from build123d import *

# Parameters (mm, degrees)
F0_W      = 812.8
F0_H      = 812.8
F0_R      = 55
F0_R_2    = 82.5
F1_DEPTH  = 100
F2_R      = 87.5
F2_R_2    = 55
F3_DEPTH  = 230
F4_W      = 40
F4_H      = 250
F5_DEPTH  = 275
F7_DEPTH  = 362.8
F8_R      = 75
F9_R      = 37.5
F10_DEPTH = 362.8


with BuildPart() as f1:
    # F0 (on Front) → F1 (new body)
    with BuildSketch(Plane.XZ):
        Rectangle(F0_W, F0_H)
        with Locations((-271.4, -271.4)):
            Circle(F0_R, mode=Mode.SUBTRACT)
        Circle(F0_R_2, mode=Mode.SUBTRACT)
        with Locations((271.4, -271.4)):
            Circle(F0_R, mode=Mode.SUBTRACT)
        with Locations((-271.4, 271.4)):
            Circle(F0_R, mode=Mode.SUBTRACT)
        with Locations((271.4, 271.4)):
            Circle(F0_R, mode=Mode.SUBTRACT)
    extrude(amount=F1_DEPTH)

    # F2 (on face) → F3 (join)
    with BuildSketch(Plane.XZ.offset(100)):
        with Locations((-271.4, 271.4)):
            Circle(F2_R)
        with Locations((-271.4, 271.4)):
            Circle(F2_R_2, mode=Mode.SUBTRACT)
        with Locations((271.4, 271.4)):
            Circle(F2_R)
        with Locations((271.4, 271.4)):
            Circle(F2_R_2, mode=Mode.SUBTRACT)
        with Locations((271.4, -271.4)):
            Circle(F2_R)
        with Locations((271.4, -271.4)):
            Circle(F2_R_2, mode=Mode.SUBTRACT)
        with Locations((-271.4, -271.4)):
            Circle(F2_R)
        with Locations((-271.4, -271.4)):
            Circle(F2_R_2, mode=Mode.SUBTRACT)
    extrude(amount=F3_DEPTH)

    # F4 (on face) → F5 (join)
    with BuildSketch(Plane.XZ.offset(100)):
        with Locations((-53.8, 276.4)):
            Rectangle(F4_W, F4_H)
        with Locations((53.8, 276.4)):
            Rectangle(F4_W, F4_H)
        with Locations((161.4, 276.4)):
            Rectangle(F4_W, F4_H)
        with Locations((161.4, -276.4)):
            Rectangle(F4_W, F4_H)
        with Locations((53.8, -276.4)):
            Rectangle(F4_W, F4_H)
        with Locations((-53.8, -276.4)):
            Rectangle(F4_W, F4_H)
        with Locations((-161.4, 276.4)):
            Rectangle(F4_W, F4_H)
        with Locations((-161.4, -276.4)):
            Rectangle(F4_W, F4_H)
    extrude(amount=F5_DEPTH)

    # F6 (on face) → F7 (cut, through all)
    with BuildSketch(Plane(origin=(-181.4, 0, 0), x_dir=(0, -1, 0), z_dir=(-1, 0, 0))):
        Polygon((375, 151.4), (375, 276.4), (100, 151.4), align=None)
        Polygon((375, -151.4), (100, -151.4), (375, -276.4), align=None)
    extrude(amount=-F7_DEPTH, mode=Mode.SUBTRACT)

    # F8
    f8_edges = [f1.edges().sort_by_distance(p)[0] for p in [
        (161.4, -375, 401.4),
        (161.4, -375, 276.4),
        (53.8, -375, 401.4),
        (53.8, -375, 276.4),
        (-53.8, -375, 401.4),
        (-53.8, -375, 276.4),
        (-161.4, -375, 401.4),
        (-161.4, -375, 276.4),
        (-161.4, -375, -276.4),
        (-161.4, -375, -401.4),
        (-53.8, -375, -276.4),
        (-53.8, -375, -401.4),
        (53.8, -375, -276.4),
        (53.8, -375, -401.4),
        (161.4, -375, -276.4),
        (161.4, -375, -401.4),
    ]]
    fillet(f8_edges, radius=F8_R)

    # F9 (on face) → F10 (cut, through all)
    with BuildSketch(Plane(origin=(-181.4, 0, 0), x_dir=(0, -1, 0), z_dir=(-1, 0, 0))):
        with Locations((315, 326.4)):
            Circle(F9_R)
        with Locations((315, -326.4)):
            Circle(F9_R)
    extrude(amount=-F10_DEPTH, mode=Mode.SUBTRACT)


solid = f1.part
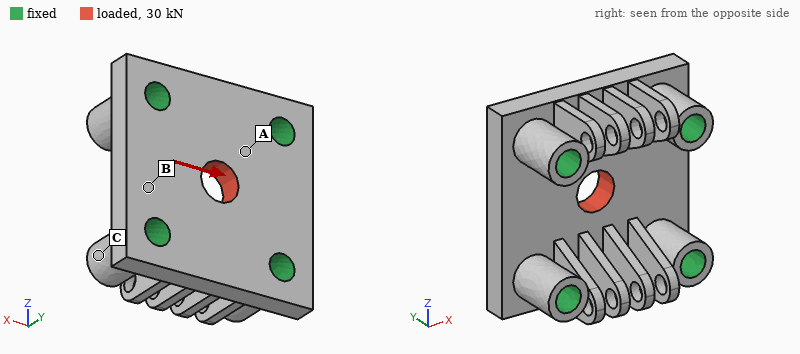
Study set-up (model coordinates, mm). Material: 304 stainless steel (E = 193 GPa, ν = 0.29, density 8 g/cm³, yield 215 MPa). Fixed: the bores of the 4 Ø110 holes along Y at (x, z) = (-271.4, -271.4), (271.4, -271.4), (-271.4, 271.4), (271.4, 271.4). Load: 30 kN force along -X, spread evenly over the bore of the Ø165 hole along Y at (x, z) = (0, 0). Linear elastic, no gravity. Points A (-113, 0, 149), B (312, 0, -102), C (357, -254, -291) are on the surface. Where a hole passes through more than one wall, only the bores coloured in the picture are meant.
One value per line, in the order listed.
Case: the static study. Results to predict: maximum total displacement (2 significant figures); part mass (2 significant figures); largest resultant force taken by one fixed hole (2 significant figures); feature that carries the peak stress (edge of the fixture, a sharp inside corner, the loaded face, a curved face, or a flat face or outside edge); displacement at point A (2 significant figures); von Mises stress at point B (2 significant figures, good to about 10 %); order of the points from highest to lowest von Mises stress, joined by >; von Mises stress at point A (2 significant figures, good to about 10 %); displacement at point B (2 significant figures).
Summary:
0.80 µm
700 kg
8.2 kN
a sharp inside corner
0.35 µm
0.20 MPa
A > B > C
0.39 MPa
0.35 µm
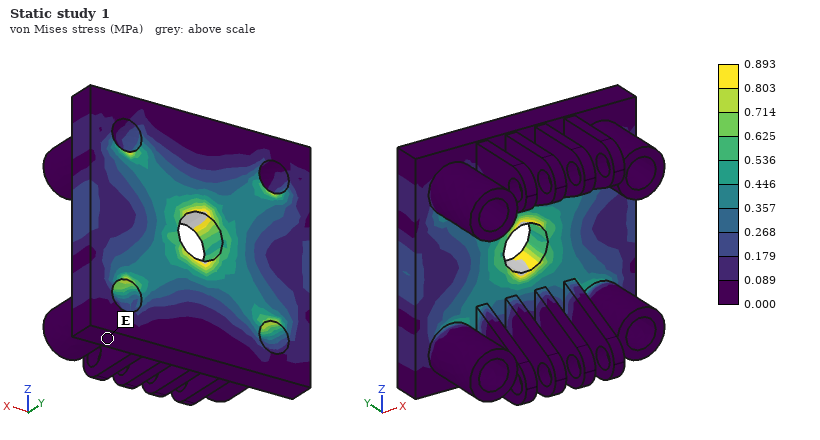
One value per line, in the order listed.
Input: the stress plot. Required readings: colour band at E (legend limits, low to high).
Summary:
0.000 to 0.089 MPa
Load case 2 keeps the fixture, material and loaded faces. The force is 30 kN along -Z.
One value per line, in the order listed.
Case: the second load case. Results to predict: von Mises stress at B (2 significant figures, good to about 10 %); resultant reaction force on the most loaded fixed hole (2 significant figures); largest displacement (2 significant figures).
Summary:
0.075 MPa
8.2 kN
0.80 µm
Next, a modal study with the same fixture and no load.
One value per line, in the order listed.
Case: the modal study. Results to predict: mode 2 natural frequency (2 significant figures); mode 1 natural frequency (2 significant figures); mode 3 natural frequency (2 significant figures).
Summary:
560 Hz
550 Hz
560 Hz
